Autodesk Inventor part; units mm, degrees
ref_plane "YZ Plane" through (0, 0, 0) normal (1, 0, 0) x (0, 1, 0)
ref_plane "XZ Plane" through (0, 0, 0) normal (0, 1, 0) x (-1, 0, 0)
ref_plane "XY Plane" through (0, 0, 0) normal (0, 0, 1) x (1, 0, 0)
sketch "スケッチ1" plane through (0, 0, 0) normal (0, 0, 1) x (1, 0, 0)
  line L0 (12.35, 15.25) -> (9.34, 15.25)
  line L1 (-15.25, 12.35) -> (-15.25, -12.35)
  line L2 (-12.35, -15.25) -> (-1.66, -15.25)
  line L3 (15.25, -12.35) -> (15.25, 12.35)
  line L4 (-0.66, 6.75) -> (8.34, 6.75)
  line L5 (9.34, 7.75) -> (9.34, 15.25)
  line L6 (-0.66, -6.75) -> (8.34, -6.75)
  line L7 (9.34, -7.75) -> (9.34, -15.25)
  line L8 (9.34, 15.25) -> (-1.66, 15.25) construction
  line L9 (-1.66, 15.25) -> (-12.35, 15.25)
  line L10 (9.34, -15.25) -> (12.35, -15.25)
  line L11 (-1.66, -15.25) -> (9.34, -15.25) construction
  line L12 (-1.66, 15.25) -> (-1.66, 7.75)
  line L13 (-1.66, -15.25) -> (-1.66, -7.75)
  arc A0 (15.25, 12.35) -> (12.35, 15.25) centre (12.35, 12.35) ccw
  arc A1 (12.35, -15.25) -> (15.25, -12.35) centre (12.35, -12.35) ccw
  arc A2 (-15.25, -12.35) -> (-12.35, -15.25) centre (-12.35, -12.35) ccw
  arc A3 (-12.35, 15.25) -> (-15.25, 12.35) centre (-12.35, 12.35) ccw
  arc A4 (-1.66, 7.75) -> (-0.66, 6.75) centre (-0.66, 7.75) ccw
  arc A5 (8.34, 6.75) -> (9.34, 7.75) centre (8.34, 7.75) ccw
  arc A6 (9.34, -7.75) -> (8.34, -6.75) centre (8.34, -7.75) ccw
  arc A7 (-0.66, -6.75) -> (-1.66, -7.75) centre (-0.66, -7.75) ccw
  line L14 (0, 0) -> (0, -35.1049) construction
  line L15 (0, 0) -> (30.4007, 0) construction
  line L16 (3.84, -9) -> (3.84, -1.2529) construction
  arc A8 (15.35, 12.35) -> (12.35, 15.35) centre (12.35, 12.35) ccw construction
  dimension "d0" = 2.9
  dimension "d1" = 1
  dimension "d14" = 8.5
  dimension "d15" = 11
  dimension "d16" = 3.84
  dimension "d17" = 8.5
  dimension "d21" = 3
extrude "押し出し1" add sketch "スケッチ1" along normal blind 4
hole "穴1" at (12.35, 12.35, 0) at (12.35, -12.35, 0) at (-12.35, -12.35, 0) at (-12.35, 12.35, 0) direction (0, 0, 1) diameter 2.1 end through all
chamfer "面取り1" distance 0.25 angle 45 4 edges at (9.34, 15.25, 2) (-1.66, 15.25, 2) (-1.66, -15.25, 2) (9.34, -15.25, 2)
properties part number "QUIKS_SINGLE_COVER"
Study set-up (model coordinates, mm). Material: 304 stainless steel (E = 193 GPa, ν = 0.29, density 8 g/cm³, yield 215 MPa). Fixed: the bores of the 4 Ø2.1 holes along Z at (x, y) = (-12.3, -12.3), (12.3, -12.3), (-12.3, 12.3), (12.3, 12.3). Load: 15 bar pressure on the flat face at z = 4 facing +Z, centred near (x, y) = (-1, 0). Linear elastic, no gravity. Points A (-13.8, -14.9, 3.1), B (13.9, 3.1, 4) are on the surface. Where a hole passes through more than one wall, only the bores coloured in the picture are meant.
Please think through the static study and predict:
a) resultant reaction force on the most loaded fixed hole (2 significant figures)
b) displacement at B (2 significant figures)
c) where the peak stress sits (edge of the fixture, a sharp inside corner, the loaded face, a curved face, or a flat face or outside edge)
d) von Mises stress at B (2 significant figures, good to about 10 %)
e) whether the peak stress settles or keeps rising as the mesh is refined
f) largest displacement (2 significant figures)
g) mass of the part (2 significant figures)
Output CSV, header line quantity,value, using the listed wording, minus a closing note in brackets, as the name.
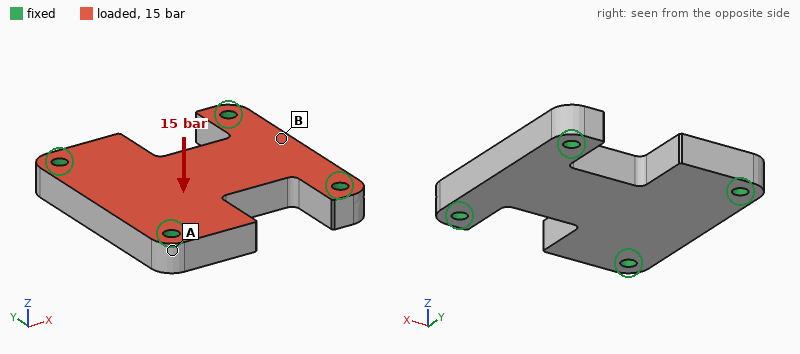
quantity,value
resultant reaction force on the most loaded fixed hole,320 N
displacement at B,2.4 µm
where the peak stress sits,edge of the fixture
von Mises stress at B,18 MPa
whether the peak stress settles or keeps rising as the mesh is refined,keeps rising
largest displacement,5.4 µm
mass of the part,23 g
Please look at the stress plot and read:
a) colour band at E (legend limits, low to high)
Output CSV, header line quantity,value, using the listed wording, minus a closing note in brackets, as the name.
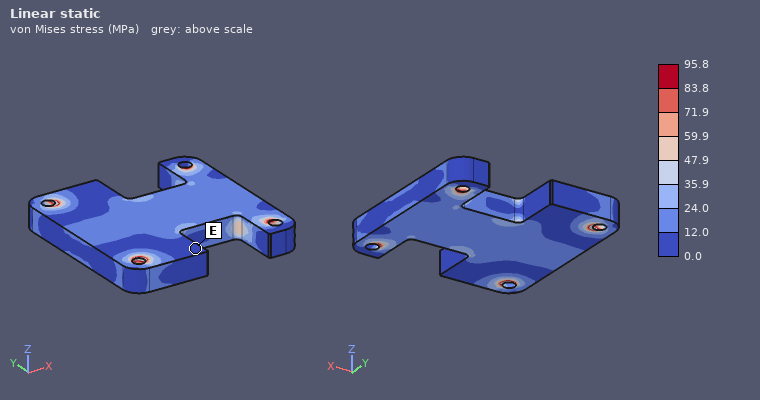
quantity,value
colour band at E,0.0 to 12.0 MPa
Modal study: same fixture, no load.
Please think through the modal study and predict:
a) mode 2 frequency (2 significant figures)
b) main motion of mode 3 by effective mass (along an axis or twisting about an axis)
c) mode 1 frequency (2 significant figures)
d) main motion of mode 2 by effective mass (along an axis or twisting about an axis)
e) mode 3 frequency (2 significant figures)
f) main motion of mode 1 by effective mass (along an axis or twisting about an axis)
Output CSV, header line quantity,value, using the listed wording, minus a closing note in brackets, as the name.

quantity,value
mode 2 frequency,29 kHz
main motion of mode 3 by effective mass,twisting about X
mode 1 frequency,17 kHz
main motion of mode 2 by effective mass,twisting about Y
mode 3 frequency,32 kHz
main motion of mode 1 by effective mass,along Z
